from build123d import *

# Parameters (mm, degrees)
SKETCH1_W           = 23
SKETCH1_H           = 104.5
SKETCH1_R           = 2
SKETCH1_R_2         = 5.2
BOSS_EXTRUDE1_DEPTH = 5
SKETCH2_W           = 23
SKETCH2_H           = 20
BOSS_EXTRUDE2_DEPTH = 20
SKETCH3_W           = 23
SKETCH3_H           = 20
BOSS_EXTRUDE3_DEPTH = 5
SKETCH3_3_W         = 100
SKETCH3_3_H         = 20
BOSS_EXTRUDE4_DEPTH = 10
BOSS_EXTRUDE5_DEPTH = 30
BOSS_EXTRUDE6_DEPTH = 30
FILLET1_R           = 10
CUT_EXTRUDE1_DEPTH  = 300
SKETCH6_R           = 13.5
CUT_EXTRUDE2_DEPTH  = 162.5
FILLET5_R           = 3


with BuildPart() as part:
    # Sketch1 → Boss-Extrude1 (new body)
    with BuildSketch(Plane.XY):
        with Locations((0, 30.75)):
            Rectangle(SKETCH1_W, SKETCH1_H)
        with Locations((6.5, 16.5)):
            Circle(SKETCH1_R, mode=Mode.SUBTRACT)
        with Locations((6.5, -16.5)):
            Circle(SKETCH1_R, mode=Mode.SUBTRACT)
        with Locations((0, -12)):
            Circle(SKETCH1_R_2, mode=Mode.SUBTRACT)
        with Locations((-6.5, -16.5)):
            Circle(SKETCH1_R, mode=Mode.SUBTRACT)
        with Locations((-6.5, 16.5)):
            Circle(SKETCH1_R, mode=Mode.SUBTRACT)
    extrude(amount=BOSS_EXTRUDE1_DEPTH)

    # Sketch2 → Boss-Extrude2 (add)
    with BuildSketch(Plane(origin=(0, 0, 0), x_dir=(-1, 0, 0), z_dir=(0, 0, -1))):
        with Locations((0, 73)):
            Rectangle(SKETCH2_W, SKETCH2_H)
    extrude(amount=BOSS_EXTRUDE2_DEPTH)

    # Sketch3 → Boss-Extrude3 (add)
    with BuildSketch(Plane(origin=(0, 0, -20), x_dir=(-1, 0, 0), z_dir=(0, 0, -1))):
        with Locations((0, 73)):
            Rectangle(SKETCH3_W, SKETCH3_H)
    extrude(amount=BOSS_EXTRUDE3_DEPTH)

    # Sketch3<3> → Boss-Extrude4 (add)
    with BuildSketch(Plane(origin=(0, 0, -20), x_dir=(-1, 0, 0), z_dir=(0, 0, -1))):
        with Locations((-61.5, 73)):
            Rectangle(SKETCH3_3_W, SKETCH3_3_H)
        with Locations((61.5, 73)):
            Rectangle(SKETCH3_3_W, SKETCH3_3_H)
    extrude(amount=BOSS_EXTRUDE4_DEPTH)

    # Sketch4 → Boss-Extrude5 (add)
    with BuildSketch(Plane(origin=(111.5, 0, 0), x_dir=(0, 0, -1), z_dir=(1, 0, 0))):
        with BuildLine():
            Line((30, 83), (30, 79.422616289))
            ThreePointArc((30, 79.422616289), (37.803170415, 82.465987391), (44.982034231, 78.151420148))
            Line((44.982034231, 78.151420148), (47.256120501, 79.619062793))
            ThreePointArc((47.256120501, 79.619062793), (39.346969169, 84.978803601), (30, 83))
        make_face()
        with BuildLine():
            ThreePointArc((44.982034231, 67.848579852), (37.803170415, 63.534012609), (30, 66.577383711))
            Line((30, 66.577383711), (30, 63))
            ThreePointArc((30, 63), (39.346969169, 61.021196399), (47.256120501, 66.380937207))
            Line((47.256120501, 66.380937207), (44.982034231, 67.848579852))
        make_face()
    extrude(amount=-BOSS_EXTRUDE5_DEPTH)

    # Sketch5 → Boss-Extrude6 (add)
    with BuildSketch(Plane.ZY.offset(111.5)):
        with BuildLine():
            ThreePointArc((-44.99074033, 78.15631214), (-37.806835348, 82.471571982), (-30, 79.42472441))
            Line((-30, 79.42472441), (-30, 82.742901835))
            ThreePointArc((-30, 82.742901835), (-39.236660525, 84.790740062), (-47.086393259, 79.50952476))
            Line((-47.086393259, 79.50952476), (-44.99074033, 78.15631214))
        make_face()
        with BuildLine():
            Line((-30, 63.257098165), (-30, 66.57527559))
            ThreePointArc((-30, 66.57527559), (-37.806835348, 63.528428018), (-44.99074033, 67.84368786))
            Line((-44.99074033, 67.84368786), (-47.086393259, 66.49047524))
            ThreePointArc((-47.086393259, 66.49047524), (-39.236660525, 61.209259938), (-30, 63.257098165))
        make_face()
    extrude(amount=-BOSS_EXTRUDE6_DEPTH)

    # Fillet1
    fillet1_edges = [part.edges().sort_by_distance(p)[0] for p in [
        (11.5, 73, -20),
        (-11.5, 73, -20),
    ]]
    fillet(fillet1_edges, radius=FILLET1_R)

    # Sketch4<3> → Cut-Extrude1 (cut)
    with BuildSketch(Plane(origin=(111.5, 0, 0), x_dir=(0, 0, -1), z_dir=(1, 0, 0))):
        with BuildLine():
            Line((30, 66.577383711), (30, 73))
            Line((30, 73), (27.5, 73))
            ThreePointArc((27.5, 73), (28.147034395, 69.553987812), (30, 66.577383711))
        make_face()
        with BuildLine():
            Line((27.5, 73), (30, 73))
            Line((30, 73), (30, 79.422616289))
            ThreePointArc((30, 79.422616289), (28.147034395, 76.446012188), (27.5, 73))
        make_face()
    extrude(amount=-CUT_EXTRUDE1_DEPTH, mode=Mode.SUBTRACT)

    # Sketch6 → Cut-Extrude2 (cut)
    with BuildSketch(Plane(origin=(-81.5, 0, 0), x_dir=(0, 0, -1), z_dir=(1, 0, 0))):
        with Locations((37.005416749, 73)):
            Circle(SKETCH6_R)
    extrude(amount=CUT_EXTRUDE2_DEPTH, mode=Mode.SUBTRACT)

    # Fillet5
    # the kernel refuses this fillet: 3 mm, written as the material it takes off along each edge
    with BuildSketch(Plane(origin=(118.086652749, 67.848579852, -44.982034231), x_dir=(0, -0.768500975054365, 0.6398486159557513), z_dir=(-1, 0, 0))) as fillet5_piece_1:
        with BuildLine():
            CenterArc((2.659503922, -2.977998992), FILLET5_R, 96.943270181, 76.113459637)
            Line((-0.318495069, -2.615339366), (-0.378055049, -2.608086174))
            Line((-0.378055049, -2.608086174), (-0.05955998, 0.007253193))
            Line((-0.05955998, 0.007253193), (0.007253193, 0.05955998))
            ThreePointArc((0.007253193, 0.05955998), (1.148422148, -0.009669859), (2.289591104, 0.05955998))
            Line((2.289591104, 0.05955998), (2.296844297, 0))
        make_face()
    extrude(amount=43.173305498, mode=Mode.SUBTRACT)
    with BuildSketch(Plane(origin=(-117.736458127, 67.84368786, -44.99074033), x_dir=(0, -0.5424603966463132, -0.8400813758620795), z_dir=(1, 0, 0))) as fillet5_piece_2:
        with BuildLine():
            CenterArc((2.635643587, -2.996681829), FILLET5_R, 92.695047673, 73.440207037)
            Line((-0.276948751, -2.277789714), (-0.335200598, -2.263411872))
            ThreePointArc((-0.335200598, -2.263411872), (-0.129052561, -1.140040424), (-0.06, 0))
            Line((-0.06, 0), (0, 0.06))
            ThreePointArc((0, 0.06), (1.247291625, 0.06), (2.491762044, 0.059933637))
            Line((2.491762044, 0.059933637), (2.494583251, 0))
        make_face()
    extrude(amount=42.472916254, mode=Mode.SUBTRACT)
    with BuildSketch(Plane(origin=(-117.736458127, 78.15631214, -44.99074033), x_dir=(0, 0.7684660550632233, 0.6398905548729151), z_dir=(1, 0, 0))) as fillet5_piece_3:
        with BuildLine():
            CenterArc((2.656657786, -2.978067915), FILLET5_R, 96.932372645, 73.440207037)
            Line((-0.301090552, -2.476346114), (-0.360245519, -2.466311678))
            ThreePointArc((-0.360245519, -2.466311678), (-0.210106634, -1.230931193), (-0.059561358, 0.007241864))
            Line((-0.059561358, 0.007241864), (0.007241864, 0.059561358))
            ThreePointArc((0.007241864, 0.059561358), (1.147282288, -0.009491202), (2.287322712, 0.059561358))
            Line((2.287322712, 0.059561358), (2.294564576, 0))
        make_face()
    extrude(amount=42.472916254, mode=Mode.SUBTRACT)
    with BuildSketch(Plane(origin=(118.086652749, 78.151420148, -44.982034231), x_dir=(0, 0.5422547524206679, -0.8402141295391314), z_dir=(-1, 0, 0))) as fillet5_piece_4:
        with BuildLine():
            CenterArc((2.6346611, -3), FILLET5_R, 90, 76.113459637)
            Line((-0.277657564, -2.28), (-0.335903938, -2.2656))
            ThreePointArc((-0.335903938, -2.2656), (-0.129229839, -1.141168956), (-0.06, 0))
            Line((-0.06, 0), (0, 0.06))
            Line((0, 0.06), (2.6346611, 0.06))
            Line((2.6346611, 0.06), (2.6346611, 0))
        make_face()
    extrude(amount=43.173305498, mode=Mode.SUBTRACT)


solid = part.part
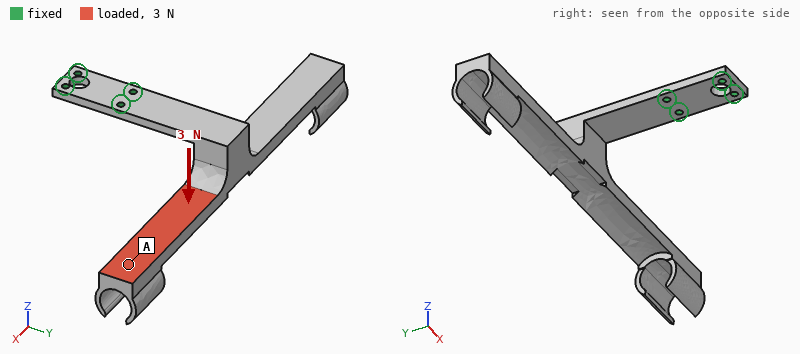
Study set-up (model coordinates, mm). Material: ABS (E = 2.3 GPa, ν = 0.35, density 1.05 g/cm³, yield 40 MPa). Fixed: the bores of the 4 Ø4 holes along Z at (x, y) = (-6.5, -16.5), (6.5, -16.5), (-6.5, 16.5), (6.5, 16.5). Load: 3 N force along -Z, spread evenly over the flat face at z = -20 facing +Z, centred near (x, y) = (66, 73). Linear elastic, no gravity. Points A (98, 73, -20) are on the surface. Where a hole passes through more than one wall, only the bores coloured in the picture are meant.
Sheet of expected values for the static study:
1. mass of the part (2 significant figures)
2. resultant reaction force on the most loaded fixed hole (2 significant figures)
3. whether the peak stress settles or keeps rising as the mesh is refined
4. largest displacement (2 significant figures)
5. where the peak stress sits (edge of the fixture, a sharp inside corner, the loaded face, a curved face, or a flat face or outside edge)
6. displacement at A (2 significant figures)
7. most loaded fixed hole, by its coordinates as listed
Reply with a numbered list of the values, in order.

1. 56 g
2. 14 N
3. keeps rising
4. 2.3 mm
5. edge of the fixture
6. 1.9 mm
7. (6.5, 16.5)
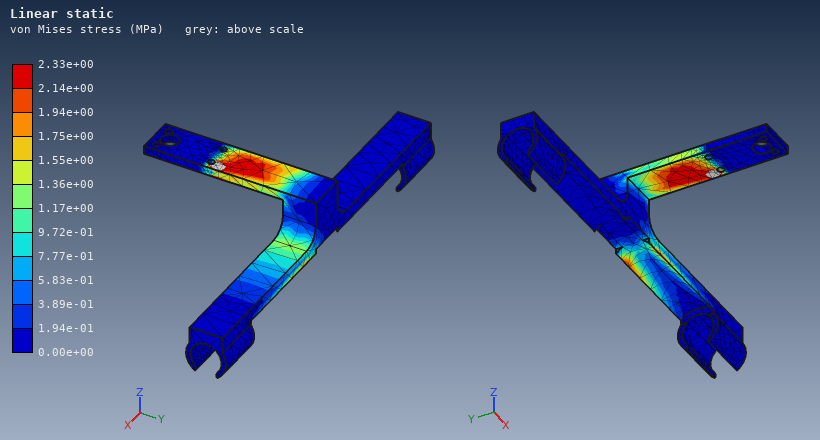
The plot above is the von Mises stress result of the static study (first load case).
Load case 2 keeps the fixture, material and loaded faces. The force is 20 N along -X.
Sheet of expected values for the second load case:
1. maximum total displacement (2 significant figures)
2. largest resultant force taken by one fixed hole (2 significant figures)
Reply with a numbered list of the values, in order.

1. 3.0 mm
2. 76 N
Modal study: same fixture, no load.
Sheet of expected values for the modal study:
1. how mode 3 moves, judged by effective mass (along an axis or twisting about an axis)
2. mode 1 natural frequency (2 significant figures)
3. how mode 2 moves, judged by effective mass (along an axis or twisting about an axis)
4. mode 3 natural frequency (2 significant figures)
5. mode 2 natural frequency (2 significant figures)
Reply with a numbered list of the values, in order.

1. along Y
2. 41 Hz
3. along Z
4. 110 Hz
5. 54 Hz
